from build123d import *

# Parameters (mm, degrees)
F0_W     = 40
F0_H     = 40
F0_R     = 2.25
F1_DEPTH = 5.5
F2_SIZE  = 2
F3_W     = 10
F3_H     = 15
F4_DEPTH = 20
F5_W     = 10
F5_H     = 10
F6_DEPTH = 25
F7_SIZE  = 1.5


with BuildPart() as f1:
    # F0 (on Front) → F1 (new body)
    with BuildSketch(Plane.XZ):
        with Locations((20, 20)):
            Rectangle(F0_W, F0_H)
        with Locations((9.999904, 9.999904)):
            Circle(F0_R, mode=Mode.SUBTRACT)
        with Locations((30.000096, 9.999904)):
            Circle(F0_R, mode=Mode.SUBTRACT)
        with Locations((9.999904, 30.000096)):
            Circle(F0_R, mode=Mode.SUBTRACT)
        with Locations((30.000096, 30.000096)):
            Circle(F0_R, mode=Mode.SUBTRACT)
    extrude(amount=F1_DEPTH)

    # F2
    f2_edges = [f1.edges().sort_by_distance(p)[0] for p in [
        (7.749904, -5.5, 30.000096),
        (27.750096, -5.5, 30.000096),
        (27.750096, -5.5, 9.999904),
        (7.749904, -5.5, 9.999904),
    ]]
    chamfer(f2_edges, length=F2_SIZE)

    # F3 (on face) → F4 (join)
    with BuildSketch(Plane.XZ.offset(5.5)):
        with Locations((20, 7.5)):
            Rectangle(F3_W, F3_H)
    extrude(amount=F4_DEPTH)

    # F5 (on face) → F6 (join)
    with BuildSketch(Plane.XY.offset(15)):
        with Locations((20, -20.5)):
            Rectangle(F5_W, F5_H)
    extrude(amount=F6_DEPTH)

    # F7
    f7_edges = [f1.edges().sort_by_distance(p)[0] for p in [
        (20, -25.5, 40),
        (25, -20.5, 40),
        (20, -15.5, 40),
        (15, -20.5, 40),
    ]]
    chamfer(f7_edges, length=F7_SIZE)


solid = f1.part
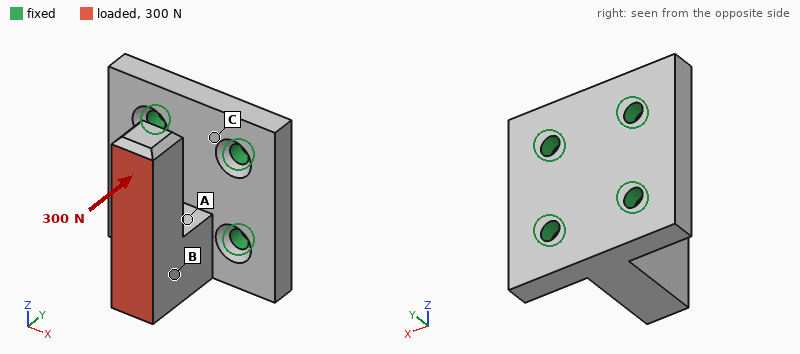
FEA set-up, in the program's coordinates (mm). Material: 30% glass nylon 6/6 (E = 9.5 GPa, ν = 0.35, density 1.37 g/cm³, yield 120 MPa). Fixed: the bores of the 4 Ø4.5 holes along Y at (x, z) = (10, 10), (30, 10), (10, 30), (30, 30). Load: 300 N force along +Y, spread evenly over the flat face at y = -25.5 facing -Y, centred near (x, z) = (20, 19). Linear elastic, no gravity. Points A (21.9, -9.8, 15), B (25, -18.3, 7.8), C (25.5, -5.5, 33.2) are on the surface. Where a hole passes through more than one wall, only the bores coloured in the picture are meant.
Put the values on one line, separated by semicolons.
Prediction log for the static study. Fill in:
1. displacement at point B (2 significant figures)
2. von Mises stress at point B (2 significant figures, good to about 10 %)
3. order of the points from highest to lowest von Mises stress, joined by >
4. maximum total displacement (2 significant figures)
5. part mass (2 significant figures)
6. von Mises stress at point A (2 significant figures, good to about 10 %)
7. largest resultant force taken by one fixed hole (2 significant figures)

0.044 mm; 5.4 MPa; A > B > C; 0.22 mm; 19 g; 11 MPa; 120 N
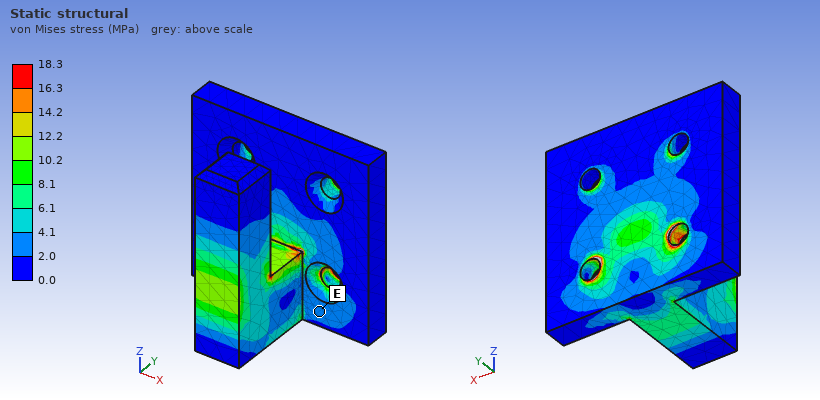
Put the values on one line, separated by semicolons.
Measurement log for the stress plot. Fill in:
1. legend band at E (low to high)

2.0 to 4.1 MPa
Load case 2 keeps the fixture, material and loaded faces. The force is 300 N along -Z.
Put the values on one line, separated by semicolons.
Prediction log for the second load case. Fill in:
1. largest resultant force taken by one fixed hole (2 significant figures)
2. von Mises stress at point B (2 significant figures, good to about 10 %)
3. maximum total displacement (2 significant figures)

200 N; 6.7 MPa; 0.33 mm
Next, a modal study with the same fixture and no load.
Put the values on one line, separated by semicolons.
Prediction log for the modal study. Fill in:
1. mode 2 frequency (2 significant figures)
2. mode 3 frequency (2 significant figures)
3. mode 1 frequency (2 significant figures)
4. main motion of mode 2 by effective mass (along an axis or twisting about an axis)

2500 Hz; 5700 Hz; 2400 Hz; along X
